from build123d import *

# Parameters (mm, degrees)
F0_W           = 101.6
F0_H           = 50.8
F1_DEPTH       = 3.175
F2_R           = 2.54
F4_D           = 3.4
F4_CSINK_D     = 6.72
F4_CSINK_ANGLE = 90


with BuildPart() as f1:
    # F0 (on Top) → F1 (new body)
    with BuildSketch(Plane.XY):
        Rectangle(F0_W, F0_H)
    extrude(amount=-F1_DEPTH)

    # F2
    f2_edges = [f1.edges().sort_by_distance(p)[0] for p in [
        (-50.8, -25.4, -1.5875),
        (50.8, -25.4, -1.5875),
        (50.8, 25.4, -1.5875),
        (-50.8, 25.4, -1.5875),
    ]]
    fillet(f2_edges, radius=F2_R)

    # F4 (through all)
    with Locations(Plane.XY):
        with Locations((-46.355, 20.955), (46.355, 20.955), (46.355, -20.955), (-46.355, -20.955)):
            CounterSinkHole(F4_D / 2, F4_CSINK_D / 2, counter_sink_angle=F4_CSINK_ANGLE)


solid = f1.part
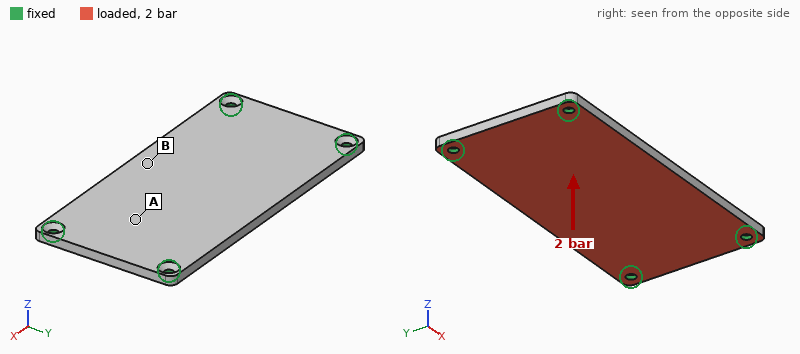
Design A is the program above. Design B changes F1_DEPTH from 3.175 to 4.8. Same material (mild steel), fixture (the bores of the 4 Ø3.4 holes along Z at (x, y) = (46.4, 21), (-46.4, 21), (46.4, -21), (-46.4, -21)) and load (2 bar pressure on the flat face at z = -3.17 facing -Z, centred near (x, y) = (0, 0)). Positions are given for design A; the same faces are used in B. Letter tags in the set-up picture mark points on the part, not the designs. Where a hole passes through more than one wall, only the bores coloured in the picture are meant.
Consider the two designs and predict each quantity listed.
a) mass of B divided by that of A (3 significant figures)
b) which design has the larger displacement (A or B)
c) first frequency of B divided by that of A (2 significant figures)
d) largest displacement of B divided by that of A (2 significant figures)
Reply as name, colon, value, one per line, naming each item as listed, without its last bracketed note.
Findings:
mass of B divided by that of A: 1.51
which design has the larger displacement: A
first frequency of B divided by that of A: 1.5
largest displacement of B divided by that of A: 0.29
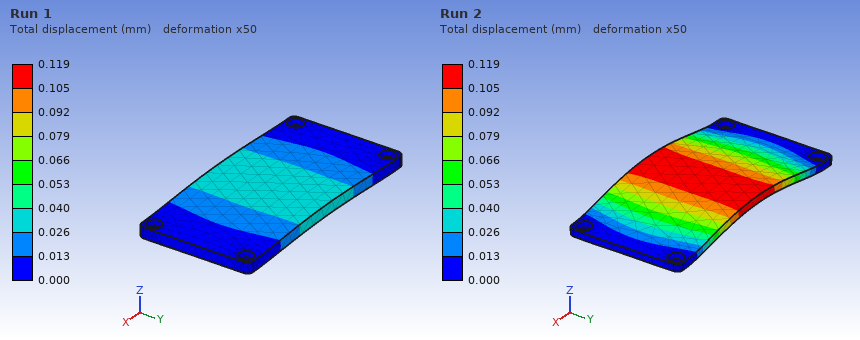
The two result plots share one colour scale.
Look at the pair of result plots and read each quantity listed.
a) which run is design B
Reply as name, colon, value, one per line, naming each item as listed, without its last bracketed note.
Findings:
which run is design B: Run 1
